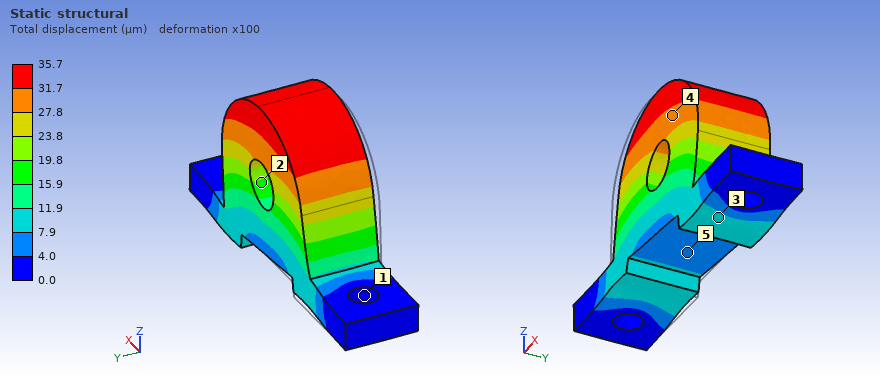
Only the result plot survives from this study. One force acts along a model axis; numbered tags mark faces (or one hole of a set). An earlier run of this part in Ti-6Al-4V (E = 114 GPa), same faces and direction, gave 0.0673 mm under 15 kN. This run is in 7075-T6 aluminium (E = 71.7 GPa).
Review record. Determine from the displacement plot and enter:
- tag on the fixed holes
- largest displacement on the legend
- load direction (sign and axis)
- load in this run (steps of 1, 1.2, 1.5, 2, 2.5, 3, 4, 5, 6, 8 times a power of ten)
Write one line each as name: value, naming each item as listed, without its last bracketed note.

tag on the fixed holes: 1
largest displacement on the legend: 35.7 µm
load direction: +X
load in this run: 5 kN
